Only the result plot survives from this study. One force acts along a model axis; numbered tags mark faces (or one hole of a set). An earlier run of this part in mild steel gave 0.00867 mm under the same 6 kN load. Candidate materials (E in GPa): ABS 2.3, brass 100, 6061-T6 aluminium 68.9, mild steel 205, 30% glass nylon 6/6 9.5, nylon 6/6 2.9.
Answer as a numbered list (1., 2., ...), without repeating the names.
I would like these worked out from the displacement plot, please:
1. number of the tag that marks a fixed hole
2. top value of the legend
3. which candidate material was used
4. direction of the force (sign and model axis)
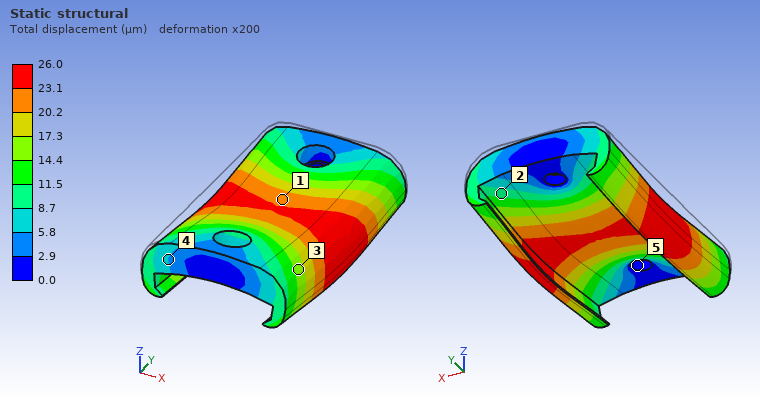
1. 5
2. 26.0 µm
3. 6061-T6 aluminium
4. -Z
